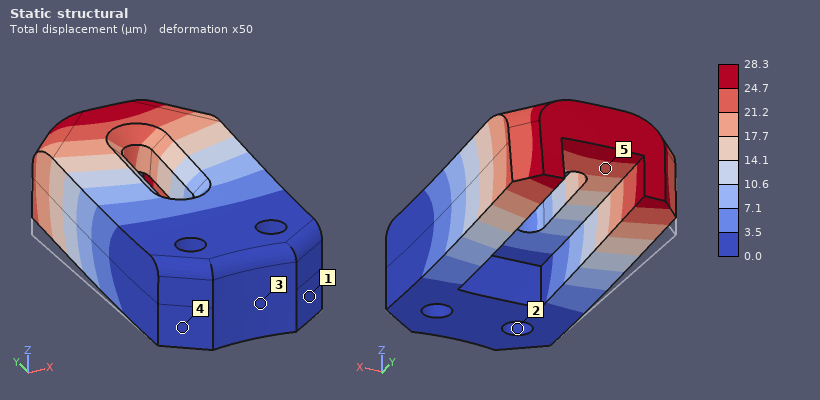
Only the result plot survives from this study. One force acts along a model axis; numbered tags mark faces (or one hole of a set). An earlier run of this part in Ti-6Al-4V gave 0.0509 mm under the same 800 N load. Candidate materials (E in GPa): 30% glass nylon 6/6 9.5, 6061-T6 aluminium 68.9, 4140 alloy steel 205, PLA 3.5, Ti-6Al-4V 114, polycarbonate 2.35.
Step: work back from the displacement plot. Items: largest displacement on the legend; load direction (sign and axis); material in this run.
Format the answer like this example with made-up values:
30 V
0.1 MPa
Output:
28.3 µm
+Z
4140 alloy steel
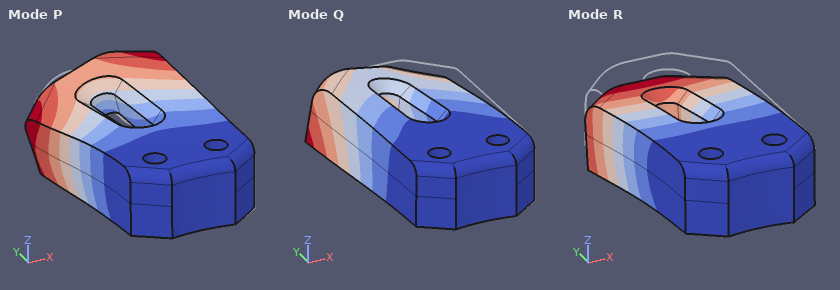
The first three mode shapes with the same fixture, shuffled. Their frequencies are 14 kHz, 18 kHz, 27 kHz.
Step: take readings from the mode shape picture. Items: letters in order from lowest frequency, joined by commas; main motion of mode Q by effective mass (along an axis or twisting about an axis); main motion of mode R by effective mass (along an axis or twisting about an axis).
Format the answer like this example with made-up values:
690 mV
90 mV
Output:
R, Q, P
along X
along Z
